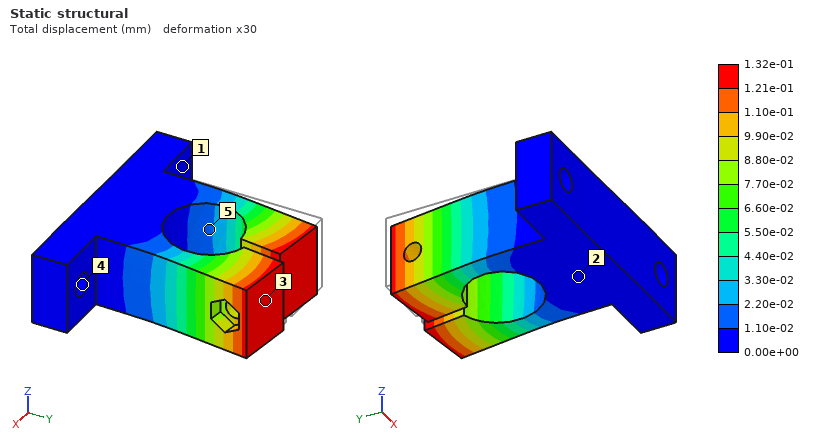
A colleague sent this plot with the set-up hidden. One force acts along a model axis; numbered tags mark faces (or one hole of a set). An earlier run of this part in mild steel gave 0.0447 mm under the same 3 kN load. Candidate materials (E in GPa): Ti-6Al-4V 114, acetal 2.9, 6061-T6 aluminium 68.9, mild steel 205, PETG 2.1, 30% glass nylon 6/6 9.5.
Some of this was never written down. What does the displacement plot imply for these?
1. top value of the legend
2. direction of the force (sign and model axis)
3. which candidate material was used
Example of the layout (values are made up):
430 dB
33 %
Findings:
1.32e-01 mm
+X
6061-T6 aluminium
